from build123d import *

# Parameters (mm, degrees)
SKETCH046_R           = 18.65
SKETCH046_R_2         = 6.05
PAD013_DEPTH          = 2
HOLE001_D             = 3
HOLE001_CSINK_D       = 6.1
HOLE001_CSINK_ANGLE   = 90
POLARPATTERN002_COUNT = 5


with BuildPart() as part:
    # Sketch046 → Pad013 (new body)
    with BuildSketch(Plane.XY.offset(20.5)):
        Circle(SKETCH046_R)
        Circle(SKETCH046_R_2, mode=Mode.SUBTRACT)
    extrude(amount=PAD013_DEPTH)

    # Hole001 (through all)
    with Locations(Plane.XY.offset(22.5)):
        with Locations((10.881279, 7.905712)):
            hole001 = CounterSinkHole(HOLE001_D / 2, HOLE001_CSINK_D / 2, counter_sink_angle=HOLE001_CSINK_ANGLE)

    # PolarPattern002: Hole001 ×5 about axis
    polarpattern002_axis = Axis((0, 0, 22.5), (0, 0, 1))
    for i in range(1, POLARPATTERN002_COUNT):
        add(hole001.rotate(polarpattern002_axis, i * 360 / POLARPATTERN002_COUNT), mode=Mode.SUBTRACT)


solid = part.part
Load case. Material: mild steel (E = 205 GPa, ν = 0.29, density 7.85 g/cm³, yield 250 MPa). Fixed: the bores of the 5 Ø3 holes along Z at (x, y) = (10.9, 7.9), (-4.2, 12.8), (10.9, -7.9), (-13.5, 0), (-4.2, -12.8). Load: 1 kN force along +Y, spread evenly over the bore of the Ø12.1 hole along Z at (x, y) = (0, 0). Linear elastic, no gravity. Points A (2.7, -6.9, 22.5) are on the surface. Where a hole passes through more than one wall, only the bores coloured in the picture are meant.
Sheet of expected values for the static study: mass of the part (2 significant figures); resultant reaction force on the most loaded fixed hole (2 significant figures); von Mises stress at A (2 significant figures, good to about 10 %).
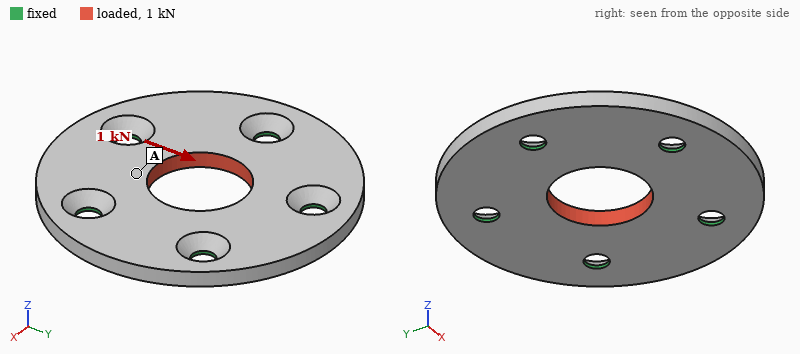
14 g
230 N
11 MPa
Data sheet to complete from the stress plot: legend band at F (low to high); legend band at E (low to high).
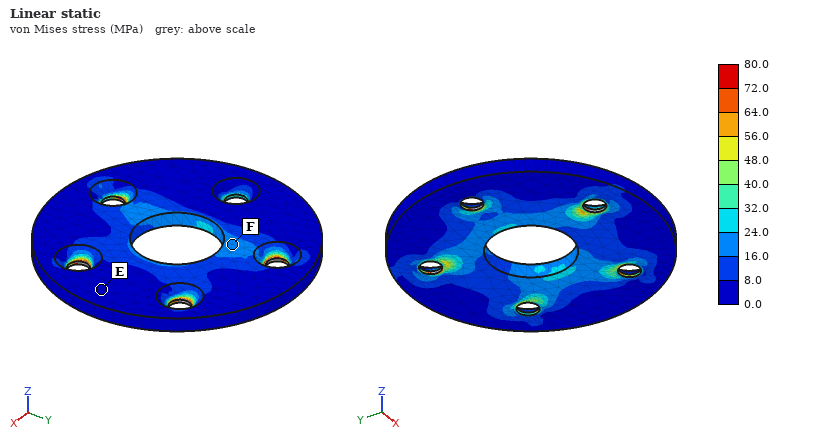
16.0 to 24.0 MPa
0.0 to 8.0 MPa
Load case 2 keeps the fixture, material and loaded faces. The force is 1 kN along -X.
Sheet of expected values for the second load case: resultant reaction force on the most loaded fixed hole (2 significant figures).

240 N
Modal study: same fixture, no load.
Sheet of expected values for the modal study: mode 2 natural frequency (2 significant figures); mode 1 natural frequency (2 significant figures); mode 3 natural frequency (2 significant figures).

19 kHz
19 kHz
20 kHz
